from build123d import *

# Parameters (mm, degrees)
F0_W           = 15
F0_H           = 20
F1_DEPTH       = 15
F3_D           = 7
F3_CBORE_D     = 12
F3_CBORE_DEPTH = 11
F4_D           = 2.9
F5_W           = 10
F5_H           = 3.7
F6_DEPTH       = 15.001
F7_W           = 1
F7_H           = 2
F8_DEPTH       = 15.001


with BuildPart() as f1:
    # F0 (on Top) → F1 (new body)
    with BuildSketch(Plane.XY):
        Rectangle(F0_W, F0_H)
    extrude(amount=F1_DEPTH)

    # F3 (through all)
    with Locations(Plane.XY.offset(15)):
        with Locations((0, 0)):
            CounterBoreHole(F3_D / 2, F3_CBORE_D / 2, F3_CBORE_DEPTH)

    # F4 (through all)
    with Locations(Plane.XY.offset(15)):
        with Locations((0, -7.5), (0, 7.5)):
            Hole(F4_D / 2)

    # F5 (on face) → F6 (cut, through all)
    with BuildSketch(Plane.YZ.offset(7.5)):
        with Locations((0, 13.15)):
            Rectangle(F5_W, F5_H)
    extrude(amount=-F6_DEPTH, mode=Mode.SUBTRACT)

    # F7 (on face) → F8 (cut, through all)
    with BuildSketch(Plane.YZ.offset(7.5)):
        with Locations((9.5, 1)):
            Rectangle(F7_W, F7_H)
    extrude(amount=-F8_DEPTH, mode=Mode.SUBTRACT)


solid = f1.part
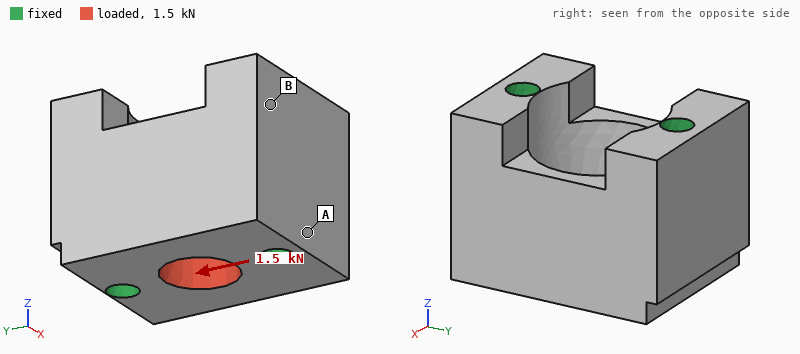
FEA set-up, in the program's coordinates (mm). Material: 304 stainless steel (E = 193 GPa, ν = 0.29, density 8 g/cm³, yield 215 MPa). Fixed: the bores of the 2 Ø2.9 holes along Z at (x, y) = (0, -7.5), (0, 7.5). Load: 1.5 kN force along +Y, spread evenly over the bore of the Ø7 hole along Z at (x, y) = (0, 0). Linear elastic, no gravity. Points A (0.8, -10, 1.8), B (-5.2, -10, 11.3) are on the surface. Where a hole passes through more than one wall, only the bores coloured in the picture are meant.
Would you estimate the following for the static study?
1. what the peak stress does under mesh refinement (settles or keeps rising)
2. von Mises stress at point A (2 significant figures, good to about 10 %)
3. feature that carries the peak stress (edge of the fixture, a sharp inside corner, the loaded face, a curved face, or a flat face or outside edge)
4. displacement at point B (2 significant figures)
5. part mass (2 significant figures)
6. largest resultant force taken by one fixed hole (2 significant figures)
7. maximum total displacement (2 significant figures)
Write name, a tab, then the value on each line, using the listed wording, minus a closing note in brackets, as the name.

what the peak stress does under mesh refinement	keeps rising
von Mises stress at point A	11 MPa
feature that carries the peak stress	edge of the fixture
displacement at point B	0.19 µm
part mass	22 g
largest resultant force taken by one fixed hole	760 N
maximum total displacement	0.86 µm
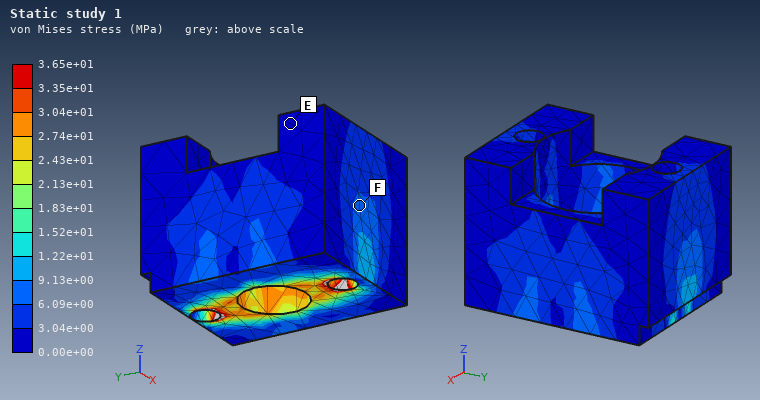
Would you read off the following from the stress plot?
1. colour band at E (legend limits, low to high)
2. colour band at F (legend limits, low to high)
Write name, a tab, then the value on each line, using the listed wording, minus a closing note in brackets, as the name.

colour band at E	0.00e+00 to 3.04e+00 MPa
colour band at F	6.09e+00 to 9.13e+00 MPa
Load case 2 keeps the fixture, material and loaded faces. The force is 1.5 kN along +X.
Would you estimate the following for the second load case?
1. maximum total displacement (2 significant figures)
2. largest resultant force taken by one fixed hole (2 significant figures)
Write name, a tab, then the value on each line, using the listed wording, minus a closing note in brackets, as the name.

maximum total displacement	1.5 µm
largest resultant force taken by one fixed hole	750 N
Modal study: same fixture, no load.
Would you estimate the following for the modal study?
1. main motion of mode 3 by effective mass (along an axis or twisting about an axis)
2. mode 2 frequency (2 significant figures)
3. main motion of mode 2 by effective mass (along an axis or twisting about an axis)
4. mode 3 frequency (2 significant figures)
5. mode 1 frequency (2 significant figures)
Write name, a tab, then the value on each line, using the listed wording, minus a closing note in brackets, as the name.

main motion of mode 3 by effective mass	twisting about Y
mode 2 frequency	60 kHz
main motion of mode 2 by effective mass	along Y
mode 3 frequency	70 kHz
mode 1 frequency	57 kHz
